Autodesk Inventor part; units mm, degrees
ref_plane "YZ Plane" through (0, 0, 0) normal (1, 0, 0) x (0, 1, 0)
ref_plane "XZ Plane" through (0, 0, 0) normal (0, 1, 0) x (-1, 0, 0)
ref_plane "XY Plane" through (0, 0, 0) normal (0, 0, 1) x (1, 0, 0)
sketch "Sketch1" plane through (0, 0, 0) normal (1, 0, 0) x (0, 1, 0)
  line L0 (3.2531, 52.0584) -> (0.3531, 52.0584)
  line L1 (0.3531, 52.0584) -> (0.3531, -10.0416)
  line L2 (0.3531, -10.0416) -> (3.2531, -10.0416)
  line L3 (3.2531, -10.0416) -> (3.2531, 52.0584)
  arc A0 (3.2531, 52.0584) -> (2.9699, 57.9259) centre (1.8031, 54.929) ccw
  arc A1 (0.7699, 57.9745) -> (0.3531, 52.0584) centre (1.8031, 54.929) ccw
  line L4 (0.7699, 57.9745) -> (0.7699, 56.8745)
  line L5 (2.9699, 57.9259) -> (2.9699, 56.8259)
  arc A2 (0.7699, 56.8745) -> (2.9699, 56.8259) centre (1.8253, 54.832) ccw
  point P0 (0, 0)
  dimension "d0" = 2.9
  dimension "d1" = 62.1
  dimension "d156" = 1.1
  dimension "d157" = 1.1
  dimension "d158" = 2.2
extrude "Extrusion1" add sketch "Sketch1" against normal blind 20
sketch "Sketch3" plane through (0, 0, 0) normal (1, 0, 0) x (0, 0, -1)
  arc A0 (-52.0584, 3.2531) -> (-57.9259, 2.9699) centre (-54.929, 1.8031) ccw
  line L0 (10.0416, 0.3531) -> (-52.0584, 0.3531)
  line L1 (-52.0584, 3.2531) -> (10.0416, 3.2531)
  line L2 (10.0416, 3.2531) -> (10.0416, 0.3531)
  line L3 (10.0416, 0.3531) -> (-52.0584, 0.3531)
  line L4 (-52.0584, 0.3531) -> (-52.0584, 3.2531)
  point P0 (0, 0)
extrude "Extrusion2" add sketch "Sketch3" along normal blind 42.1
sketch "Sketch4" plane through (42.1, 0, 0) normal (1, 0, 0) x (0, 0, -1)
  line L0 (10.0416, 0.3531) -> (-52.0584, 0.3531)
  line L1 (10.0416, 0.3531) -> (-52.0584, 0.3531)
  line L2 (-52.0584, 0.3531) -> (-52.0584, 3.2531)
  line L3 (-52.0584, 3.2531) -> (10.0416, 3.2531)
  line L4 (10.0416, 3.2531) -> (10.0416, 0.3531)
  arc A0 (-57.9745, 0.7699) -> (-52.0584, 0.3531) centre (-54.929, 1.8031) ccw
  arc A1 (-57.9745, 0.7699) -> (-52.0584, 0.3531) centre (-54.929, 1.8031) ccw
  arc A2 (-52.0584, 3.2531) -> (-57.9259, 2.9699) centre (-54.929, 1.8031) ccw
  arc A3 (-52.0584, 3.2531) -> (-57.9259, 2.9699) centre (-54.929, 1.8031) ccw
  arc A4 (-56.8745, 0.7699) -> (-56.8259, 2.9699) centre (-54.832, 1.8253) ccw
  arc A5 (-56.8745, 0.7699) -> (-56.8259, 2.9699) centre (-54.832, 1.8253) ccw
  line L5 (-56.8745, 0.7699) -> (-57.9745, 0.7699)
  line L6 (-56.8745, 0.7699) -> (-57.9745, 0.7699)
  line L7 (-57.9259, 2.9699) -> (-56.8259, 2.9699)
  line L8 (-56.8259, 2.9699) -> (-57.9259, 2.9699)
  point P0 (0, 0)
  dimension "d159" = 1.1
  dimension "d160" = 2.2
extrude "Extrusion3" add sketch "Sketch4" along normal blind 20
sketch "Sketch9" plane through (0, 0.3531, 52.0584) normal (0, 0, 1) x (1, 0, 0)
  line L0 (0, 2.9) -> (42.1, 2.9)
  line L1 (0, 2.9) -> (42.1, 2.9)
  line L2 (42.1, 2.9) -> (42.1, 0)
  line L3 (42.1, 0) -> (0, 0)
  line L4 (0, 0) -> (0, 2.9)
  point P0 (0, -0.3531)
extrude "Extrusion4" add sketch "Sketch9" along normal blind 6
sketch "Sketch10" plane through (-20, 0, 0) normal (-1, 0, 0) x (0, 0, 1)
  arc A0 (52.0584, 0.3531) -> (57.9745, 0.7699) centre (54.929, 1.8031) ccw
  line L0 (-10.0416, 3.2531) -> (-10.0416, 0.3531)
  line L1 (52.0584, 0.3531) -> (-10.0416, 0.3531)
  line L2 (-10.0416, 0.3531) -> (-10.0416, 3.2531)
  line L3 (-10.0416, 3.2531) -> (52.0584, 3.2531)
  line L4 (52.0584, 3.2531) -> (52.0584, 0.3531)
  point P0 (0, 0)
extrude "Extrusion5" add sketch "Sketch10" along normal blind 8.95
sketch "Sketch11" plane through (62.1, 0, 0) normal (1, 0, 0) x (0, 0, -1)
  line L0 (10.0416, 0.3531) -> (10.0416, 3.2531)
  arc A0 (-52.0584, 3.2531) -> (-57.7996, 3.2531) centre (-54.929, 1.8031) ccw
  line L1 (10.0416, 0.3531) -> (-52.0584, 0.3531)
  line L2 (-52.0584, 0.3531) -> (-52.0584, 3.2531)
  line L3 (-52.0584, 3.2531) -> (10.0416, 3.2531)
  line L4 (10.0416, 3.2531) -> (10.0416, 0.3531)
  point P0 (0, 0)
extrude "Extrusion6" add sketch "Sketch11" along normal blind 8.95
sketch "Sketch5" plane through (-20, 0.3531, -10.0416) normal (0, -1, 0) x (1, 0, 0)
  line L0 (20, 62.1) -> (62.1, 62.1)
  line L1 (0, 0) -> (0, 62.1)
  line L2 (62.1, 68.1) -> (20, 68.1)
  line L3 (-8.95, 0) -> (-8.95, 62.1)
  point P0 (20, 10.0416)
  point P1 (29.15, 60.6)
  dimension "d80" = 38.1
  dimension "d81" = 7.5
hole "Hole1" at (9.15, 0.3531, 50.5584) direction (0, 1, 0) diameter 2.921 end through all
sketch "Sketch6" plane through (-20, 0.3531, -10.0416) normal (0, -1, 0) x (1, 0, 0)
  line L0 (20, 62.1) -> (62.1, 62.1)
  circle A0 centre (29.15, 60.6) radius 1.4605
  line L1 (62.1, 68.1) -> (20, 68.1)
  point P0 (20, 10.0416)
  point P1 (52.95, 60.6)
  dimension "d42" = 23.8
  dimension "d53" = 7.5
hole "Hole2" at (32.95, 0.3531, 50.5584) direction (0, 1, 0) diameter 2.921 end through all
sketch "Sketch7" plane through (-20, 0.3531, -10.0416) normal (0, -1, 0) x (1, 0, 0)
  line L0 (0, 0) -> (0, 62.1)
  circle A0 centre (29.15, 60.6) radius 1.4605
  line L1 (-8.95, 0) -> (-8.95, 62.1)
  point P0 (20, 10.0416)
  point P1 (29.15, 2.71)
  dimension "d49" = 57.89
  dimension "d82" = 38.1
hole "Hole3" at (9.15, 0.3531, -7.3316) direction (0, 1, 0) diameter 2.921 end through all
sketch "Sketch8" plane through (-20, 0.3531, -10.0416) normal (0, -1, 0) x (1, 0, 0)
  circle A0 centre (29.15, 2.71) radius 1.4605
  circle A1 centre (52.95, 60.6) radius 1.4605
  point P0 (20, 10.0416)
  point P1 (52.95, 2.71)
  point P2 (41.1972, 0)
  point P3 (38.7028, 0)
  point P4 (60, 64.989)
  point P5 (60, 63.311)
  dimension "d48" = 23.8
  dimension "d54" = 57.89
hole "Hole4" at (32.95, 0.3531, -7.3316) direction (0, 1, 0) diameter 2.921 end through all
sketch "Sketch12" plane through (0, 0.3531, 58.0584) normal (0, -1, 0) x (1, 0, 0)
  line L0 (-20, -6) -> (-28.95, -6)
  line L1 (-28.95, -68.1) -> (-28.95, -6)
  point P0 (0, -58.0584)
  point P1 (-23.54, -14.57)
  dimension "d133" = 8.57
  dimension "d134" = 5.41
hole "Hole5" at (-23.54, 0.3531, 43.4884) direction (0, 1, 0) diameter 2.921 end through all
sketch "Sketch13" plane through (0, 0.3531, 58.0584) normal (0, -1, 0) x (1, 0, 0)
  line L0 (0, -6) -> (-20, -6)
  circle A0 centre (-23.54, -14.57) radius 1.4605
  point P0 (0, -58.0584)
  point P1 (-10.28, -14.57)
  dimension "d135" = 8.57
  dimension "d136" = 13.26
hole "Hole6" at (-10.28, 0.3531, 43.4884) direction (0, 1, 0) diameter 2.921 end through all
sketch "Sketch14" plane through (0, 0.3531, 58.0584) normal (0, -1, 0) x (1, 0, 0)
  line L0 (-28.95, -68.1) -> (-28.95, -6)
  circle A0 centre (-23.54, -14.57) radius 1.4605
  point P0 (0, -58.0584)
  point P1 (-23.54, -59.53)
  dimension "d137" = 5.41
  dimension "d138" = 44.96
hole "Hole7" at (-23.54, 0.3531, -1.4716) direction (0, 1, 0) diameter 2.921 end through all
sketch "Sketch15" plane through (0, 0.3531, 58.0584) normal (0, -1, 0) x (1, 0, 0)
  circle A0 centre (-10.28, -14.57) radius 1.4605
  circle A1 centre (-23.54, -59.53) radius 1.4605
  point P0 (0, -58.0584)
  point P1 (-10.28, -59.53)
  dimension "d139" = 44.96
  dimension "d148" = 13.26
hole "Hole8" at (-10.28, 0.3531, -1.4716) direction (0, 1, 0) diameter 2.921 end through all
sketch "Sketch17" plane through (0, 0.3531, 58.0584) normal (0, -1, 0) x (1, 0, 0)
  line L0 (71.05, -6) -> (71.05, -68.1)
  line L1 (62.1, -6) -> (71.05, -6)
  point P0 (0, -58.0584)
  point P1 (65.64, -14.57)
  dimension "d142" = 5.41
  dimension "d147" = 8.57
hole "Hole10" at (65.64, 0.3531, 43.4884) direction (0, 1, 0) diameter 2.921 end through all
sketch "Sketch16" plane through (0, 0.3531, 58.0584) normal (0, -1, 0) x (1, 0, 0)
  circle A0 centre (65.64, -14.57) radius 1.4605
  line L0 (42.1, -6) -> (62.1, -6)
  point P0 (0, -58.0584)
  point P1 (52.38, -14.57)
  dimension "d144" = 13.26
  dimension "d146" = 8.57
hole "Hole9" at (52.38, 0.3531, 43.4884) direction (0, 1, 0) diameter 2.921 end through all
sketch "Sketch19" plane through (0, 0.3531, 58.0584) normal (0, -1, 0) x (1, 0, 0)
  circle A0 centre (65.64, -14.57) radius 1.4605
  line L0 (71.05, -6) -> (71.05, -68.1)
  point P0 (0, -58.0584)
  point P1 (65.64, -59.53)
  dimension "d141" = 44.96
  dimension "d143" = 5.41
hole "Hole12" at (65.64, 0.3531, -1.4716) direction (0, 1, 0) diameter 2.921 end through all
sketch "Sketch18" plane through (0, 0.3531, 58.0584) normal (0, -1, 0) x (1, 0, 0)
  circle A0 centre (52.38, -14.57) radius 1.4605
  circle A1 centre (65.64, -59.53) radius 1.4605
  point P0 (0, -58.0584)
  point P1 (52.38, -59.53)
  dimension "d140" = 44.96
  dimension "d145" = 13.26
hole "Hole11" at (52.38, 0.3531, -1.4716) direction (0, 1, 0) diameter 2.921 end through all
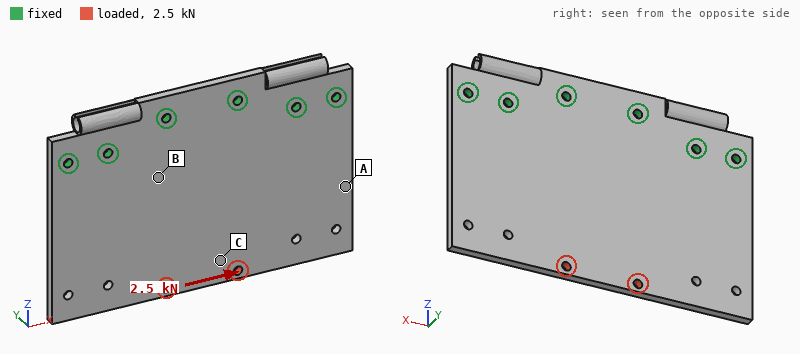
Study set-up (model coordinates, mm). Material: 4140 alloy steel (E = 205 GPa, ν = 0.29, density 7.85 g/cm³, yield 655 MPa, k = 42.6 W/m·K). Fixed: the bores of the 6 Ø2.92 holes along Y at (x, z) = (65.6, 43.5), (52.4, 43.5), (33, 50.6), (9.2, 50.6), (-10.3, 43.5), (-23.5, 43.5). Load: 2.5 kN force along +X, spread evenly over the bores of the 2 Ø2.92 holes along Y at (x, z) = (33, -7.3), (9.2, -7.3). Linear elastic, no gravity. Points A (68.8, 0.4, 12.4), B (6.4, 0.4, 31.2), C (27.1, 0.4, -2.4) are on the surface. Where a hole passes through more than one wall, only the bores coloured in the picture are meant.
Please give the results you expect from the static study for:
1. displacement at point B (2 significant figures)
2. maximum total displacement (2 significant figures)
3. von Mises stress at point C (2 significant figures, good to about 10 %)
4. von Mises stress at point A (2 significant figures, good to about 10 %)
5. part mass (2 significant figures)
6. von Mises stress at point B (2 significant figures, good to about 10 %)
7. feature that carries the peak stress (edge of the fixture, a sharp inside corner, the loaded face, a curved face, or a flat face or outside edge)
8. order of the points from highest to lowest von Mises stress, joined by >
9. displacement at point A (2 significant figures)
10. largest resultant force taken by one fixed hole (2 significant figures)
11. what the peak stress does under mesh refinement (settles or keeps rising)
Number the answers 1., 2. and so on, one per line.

1. 2.1 µm
2. 11 µm
3. 26 MPa
4. 7.3 MPa
5. 150 g
6. 17 MPa
7. edge of the fixture
8. C > B > A
9. 6.3 µm
10. 1.1 kN
11. keeps rising
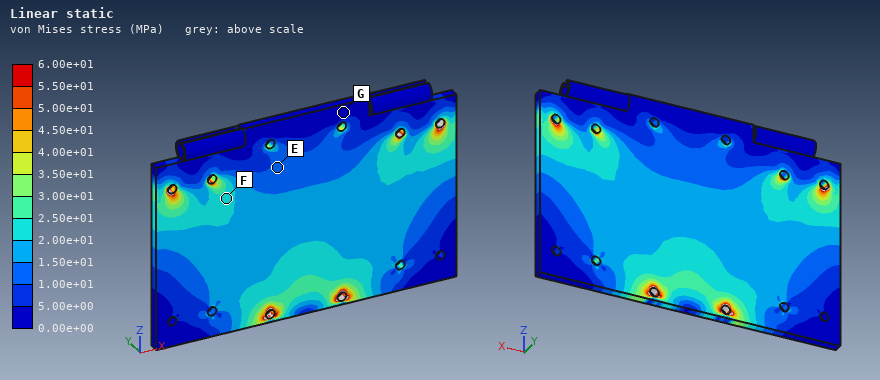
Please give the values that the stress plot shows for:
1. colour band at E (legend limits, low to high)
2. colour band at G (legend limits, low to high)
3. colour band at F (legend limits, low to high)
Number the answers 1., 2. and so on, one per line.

1. 1.00e+01 to 1.50e+01 MPa
2. 0.00e+00 to 5.00e+00 MPa
3. 2.00e+01 to 2.50e+01 MPa
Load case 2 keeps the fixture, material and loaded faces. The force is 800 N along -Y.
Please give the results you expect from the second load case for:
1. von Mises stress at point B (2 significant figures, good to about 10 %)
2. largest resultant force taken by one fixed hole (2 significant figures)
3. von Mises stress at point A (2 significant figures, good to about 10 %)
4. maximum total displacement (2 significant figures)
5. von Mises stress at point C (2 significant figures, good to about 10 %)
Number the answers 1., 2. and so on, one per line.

1. 200 MPa
2. 690 N
3. 120 MPa
4. 1.2 mm
5. 110 MPa
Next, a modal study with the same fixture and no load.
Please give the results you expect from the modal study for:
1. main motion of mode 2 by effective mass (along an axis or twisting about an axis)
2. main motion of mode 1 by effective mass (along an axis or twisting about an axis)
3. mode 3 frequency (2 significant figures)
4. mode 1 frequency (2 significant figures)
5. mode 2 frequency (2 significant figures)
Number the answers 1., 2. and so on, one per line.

1. twisting about Z
2. along Y
3. 2600 Hz
4. 790 Hz
5. 1400 Hz
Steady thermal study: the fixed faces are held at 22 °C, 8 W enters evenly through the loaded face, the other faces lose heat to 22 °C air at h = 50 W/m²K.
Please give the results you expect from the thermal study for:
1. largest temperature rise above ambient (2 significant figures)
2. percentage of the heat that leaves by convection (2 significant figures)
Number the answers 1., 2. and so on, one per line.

1. 38 K
2. 65 %
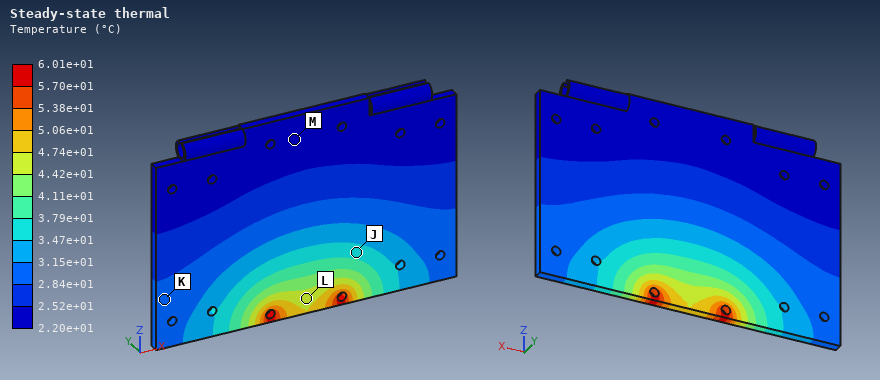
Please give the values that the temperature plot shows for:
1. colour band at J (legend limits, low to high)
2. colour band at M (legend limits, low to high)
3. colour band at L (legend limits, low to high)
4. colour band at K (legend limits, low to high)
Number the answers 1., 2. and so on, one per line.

1. 3.47e+01 to 3.79e+01 °C
2. 2.20e+01 to 2.52e+01 °C
3. 4.42e+01 to 4.74e+01 °C
4. 2.84e+01 to 3.15e+01 °C
